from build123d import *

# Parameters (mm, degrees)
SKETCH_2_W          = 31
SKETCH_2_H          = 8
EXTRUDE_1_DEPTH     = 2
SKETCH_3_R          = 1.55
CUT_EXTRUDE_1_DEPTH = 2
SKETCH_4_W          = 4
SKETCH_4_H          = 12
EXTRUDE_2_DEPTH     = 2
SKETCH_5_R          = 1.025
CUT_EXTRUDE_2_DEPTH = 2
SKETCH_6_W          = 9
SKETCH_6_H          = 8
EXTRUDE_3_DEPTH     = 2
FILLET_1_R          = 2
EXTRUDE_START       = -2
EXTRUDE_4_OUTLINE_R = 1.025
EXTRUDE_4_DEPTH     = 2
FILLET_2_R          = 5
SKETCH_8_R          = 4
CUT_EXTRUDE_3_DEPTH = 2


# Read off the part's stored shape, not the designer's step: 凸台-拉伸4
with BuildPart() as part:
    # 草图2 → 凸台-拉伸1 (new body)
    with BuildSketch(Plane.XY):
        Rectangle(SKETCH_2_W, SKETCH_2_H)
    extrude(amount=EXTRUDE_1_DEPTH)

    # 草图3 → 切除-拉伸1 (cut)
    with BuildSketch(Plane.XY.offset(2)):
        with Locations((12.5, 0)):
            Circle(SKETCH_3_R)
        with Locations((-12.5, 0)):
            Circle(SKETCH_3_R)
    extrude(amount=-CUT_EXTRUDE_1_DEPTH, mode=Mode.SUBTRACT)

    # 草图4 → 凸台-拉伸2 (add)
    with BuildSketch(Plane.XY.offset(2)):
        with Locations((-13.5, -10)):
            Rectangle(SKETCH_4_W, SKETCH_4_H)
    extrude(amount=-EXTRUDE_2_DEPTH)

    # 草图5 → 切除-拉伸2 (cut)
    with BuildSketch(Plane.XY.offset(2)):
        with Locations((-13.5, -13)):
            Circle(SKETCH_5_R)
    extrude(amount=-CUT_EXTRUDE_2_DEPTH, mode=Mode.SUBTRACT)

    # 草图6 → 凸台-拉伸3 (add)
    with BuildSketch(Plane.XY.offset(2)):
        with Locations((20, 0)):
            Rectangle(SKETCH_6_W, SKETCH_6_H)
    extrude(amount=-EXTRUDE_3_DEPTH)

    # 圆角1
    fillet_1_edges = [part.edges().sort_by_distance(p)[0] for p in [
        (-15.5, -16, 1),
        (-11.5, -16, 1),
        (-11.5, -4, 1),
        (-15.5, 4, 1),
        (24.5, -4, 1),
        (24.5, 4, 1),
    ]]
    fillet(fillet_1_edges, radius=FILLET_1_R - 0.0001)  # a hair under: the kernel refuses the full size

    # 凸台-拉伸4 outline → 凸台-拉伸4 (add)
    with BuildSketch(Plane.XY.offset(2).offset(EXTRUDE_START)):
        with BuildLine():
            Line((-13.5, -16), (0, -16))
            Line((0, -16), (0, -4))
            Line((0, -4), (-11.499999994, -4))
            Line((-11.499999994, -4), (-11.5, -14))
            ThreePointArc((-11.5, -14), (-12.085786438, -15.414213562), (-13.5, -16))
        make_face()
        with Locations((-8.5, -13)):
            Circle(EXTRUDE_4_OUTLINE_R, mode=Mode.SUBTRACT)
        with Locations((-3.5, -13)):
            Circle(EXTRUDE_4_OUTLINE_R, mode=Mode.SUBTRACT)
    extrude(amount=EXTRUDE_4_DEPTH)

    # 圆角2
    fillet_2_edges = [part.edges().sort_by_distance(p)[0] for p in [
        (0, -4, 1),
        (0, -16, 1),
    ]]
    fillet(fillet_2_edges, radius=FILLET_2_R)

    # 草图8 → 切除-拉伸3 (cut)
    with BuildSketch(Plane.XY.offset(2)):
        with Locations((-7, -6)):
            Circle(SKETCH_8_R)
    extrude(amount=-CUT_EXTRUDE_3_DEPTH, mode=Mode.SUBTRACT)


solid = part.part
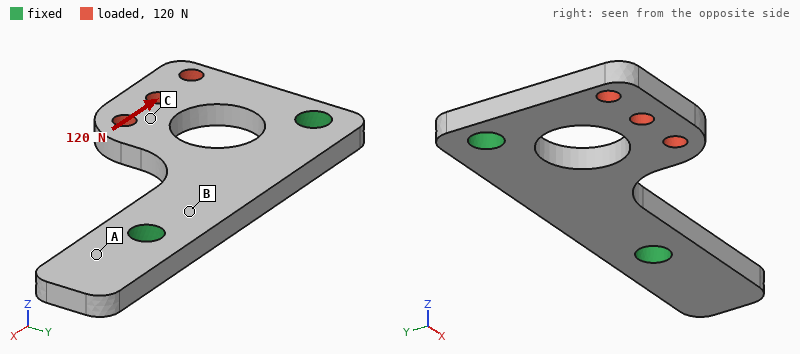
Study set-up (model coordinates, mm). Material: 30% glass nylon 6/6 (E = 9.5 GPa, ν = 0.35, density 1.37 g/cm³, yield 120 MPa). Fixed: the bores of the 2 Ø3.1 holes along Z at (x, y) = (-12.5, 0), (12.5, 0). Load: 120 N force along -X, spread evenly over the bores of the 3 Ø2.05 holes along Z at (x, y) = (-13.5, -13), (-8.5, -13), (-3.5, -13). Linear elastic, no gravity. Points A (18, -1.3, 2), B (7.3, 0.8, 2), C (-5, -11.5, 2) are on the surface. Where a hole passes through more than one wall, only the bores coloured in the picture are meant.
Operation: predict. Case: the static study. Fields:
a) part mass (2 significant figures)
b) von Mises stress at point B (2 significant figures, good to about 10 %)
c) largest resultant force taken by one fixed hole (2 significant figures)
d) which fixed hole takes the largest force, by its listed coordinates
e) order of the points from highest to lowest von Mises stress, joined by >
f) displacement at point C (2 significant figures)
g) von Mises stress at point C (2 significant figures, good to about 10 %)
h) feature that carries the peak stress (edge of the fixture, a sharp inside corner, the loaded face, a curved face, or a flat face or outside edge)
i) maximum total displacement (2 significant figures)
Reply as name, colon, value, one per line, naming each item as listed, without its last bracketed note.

part mass: 1.2 g
von Mises stress at point B: 8.4 MPa
largest resultant force taken by one fixed hole: 90 N
which fixed hole takes the largest force, by its listed coordinates: (-12.5, 0)
order of the points from highest to lowest von Mises stress, joined by >: C > B > A
displacement at point C: 50 µm
von Mises stress at point C: 14 MPa
feature that carries the peak stress: a curved face
maximum total displacement: 67 µm
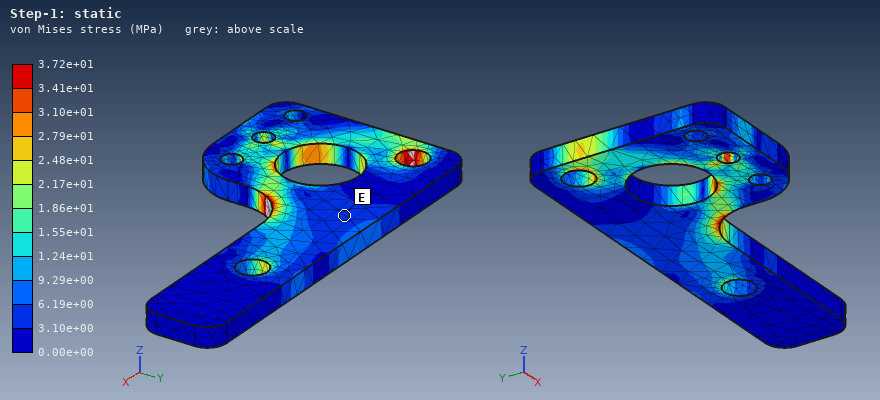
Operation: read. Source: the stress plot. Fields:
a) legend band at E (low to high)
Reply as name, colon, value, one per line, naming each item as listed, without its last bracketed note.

legend band at E: 3.10e+00 to 6.19e+00 MPa
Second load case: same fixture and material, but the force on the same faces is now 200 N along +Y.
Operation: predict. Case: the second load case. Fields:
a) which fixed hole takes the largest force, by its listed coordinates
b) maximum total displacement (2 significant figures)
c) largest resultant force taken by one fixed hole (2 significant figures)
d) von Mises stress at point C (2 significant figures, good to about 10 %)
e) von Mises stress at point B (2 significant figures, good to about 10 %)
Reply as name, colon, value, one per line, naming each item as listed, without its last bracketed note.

which fixed hole takes the largest force, by its listed coordinates: (-12.5, 0)
maximum total displacement: 28 µm
largest resultant force taken by one fixed hole: 160 N
von Mises stress at point C: 5.0 MPa
von Mises stress at point B: 5.7 MPa
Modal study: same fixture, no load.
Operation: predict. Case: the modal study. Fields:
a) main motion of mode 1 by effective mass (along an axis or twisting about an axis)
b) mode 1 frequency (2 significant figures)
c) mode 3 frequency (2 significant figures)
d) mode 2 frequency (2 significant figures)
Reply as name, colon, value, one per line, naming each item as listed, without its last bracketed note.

main motion of mode 1 by effective mass: along Z
mode 1 frequency: 3000 Hz
mode 3 frequency: 7100 Hz
mode 2 frequency: 7100 Hz
